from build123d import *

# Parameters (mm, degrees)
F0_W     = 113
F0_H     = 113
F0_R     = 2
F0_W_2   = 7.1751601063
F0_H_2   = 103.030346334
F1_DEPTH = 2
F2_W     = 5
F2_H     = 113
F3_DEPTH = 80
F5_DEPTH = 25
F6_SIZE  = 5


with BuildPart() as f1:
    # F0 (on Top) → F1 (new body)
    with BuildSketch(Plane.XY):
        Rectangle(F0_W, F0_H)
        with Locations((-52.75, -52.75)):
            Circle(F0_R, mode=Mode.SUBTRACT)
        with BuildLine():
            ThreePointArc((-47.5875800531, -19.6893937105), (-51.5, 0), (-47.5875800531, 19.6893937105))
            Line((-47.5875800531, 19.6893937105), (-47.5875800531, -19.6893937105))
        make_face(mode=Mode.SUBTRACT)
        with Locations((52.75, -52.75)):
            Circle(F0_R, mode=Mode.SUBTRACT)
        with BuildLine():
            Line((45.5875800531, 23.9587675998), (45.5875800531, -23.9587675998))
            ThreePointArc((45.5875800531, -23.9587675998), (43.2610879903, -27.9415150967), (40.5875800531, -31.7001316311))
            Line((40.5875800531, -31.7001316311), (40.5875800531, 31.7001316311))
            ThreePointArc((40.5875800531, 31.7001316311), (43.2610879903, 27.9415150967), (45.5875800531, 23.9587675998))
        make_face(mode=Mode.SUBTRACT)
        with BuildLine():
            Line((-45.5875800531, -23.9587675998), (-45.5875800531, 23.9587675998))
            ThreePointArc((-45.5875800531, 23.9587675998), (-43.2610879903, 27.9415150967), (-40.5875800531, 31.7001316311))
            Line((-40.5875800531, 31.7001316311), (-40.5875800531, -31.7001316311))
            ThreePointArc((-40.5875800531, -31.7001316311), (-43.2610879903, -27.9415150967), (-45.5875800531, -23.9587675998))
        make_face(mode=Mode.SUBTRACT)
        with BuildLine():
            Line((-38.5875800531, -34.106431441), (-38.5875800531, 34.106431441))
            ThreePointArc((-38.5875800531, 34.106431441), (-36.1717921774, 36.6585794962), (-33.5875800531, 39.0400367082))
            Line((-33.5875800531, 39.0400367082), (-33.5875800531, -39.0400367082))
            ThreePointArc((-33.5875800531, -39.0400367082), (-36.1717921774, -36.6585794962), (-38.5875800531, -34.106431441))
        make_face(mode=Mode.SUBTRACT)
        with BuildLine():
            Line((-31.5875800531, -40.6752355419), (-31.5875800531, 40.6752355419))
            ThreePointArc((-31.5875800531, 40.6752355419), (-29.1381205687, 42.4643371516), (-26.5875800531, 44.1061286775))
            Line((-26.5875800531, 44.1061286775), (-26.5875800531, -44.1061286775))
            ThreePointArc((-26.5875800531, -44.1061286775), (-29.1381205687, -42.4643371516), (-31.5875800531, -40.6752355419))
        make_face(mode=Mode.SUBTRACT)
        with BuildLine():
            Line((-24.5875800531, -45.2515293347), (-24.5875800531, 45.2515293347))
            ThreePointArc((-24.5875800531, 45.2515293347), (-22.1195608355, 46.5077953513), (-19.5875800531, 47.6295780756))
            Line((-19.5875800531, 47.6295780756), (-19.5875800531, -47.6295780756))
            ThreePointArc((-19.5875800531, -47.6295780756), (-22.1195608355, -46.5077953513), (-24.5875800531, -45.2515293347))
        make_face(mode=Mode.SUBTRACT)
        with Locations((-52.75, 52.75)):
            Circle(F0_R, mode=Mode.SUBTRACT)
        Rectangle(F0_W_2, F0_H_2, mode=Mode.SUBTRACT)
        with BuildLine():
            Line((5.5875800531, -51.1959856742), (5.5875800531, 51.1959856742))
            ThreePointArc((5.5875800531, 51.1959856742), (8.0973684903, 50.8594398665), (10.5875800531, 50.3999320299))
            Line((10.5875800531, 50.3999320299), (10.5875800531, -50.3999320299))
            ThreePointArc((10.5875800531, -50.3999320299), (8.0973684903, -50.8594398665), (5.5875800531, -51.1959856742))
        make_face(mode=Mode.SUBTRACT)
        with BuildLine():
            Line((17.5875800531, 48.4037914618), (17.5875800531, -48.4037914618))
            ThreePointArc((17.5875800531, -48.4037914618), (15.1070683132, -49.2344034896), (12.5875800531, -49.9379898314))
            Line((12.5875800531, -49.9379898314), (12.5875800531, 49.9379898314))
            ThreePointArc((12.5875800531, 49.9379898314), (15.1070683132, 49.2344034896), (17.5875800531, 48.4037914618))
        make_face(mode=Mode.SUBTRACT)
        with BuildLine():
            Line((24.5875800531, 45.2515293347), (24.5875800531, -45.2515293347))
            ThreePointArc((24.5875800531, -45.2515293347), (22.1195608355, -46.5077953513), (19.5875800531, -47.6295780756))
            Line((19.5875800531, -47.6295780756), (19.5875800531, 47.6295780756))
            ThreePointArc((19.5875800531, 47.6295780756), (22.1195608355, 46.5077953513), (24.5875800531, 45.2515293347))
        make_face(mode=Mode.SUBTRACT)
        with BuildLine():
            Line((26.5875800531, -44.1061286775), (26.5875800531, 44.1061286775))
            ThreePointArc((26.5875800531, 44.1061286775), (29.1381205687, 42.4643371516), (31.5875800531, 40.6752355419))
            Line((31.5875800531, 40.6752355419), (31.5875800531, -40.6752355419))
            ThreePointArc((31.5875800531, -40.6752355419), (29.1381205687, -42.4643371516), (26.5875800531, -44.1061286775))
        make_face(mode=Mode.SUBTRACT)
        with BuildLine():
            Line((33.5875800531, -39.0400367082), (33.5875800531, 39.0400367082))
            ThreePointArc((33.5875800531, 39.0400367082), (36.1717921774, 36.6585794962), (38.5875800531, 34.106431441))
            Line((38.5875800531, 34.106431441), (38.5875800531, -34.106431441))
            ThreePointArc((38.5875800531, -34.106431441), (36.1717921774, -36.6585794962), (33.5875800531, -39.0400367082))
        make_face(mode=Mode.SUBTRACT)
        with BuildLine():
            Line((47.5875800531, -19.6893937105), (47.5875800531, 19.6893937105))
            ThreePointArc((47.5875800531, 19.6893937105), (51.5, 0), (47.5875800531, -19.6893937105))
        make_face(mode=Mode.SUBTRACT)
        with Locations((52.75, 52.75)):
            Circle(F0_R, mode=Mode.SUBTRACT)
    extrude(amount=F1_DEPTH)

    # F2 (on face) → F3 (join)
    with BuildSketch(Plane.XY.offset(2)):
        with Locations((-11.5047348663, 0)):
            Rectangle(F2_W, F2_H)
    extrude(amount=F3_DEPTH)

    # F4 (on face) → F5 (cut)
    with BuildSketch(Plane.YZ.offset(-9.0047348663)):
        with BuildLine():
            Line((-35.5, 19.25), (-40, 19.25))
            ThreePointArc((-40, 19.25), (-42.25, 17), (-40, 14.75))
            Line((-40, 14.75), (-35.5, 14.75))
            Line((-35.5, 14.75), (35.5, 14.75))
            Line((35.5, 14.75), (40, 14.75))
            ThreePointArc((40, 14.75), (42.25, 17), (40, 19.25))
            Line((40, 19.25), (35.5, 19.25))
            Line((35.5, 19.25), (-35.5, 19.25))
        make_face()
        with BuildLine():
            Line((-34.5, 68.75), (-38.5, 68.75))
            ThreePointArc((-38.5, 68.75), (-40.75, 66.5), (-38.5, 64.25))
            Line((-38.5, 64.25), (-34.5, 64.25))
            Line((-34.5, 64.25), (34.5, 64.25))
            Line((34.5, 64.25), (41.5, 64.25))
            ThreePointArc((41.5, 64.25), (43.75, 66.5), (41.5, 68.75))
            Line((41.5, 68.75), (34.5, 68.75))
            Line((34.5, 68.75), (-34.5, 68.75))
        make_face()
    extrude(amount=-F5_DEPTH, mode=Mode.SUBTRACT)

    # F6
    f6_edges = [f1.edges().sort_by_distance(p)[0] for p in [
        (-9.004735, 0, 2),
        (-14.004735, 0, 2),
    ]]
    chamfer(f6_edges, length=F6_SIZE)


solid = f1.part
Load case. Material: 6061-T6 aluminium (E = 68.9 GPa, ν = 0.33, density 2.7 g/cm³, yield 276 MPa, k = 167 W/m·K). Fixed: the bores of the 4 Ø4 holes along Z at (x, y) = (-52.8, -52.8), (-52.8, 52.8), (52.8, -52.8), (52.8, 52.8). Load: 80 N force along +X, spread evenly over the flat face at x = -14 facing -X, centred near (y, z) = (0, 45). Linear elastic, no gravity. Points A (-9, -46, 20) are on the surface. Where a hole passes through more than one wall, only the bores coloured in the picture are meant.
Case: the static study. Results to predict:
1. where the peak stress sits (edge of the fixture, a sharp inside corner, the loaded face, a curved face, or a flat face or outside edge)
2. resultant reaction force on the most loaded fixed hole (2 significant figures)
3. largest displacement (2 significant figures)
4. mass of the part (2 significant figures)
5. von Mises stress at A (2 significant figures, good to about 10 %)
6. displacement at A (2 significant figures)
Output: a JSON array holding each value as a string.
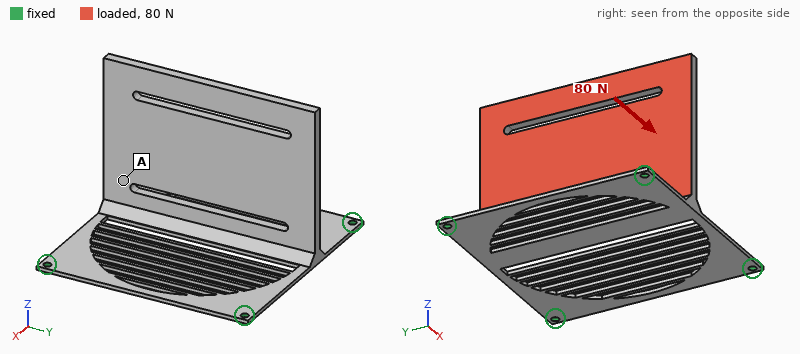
["a flat face or outside edge", "36 N", "1.9 mm", "160 g", "16 MPa", "0.52 mm"]
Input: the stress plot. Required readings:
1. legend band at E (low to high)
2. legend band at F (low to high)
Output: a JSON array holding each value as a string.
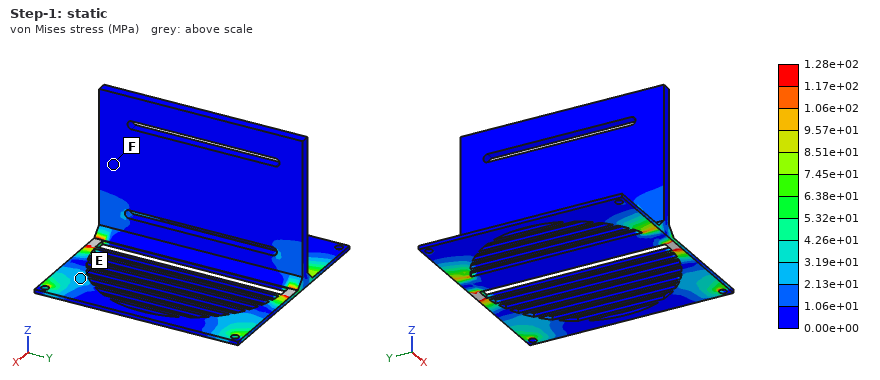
["2.13e+01 to 3.19e+01 MPa", "0.00e+00 to 1.06e+01 MPa"]
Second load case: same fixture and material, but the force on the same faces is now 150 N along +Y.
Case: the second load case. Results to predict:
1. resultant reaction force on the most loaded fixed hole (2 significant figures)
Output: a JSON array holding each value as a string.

["85 N"]
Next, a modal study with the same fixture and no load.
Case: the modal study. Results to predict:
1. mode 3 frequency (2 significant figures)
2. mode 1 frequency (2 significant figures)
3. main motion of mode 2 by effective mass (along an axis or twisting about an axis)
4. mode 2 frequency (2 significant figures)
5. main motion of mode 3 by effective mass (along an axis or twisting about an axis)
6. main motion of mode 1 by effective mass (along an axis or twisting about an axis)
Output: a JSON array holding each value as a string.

["290 Hz", "120 Hz", "along Y", "270 Hz", "along Z", "along X"]
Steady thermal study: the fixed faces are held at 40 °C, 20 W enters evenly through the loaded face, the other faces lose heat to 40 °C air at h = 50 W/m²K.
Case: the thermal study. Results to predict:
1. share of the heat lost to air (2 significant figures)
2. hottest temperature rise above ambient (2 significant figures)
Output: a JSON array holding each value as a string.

["82 %", "24 K"]
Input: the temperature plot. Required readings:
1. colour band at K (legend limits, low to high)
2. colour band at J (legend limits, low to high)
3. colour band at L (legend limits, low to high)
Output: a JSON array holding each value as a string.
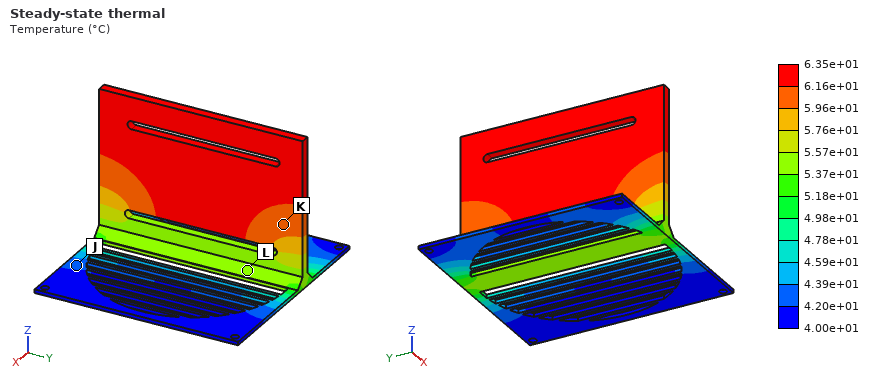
["5.96e+01 to 6.16e+01 °C", "4.20e+01 to 4.39e+01 °C", "5.37e+01 to 5.57e+01 °C"]
